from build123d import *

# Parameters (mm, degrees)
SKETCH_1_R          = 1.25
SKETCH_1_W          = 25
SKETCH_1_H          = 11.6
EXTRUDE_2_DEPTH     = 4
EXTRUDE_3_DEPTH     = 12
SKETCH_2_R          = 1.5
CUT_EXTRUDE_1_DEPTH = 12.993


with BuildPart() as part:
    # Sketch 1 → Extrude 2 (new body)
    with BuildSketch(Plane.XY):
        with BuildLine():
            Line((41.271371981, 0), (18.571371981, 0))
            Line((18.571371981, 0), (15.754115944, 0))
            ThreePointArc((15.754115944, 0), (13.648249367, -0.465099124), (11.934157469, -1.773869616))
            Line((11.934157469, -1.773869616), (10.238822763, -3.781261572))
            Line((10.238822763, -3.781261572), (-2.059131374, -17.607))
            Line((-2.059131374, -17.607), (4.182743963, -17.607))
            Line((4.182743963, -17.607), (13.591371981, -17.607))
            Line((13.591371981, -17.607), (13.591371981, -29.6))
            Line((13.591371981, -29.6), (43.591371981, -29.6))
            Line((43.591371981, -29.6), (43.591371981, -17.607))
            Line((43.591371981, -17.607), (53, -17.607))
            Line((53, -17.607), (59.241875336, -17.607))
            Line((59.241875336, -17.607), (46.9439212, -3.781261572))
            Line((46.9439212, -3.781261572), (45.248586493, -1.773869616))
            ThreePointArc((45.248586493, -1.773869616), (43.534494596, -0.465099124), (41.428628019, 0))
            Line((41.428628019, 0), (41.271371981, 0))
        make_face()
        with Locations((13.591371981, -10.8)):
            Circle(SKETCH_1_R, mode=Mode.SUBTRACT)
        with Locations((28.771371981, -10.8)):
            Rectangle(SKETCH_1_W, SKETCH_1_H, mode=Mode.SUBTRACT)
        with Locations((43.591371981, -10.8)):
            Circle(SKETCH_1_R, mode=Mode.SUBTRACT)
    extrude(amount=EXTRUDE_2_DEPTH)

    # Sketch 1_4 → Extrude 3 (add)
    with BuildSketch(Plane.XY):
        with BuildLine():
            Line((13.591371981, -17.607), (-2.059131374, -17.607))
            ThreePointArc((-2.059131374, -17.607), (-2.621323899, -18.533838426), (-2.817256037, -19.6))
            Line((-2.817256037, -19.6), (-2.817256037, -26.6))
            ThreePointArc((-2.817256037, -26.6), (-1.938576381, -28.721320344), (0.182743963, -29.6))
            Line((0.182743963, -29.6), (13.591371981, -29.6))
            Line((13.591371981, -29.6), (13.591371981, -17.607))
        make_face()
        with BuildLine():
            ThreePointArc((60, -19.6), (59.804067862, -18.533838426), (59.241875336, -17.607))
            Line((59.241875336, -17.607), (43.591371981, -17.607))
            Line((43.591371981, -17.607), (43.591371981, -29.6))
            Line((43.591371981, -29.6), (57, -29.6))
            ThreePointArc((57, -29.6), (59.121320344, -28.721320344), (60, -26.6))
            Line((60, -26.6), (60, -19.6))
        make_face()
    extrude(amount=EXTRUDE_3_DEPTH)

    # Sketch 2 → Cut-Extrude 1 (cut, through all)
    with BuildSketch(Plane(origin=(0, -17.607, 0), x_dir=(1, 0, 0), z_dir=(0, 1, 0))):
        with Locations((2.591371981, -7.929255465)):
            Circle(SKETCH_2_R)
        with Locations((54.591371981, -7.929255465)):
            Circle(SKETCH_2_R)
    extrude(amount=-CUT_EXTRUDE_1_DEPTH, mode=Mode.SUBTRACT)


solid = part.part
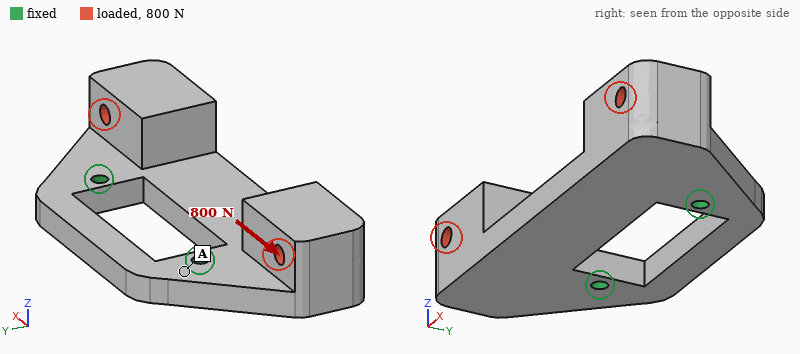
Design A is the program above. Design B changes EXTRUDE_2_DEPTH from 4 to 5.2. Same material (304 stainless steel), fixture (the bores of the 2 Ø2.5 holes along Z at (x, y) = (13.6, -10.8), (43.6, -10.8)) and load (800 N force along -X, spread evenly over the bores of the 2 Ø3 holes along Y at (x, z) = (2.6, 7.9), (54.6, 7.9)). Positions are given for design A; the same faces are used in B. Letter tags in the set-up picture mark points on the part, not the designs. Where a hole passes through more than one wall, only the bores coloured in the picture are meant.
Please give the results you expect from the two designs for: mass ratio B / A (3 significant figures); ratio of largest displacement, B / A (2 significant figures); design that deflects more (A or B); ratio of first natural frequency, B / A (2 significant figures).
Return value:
1.13
0.52
A
1.4
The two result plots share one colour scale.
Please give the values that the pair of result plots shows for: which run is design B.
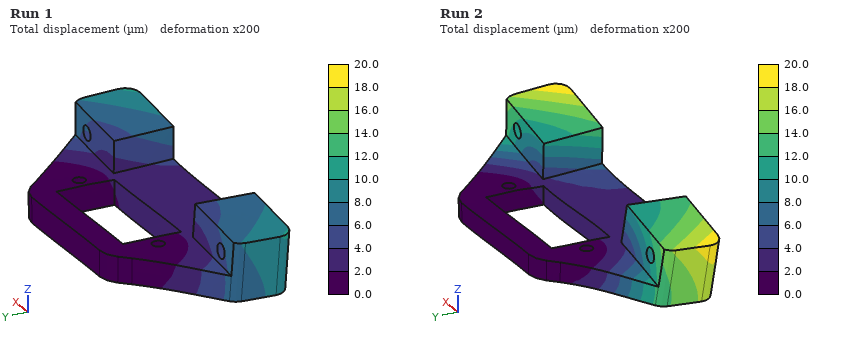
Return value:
Run 1
